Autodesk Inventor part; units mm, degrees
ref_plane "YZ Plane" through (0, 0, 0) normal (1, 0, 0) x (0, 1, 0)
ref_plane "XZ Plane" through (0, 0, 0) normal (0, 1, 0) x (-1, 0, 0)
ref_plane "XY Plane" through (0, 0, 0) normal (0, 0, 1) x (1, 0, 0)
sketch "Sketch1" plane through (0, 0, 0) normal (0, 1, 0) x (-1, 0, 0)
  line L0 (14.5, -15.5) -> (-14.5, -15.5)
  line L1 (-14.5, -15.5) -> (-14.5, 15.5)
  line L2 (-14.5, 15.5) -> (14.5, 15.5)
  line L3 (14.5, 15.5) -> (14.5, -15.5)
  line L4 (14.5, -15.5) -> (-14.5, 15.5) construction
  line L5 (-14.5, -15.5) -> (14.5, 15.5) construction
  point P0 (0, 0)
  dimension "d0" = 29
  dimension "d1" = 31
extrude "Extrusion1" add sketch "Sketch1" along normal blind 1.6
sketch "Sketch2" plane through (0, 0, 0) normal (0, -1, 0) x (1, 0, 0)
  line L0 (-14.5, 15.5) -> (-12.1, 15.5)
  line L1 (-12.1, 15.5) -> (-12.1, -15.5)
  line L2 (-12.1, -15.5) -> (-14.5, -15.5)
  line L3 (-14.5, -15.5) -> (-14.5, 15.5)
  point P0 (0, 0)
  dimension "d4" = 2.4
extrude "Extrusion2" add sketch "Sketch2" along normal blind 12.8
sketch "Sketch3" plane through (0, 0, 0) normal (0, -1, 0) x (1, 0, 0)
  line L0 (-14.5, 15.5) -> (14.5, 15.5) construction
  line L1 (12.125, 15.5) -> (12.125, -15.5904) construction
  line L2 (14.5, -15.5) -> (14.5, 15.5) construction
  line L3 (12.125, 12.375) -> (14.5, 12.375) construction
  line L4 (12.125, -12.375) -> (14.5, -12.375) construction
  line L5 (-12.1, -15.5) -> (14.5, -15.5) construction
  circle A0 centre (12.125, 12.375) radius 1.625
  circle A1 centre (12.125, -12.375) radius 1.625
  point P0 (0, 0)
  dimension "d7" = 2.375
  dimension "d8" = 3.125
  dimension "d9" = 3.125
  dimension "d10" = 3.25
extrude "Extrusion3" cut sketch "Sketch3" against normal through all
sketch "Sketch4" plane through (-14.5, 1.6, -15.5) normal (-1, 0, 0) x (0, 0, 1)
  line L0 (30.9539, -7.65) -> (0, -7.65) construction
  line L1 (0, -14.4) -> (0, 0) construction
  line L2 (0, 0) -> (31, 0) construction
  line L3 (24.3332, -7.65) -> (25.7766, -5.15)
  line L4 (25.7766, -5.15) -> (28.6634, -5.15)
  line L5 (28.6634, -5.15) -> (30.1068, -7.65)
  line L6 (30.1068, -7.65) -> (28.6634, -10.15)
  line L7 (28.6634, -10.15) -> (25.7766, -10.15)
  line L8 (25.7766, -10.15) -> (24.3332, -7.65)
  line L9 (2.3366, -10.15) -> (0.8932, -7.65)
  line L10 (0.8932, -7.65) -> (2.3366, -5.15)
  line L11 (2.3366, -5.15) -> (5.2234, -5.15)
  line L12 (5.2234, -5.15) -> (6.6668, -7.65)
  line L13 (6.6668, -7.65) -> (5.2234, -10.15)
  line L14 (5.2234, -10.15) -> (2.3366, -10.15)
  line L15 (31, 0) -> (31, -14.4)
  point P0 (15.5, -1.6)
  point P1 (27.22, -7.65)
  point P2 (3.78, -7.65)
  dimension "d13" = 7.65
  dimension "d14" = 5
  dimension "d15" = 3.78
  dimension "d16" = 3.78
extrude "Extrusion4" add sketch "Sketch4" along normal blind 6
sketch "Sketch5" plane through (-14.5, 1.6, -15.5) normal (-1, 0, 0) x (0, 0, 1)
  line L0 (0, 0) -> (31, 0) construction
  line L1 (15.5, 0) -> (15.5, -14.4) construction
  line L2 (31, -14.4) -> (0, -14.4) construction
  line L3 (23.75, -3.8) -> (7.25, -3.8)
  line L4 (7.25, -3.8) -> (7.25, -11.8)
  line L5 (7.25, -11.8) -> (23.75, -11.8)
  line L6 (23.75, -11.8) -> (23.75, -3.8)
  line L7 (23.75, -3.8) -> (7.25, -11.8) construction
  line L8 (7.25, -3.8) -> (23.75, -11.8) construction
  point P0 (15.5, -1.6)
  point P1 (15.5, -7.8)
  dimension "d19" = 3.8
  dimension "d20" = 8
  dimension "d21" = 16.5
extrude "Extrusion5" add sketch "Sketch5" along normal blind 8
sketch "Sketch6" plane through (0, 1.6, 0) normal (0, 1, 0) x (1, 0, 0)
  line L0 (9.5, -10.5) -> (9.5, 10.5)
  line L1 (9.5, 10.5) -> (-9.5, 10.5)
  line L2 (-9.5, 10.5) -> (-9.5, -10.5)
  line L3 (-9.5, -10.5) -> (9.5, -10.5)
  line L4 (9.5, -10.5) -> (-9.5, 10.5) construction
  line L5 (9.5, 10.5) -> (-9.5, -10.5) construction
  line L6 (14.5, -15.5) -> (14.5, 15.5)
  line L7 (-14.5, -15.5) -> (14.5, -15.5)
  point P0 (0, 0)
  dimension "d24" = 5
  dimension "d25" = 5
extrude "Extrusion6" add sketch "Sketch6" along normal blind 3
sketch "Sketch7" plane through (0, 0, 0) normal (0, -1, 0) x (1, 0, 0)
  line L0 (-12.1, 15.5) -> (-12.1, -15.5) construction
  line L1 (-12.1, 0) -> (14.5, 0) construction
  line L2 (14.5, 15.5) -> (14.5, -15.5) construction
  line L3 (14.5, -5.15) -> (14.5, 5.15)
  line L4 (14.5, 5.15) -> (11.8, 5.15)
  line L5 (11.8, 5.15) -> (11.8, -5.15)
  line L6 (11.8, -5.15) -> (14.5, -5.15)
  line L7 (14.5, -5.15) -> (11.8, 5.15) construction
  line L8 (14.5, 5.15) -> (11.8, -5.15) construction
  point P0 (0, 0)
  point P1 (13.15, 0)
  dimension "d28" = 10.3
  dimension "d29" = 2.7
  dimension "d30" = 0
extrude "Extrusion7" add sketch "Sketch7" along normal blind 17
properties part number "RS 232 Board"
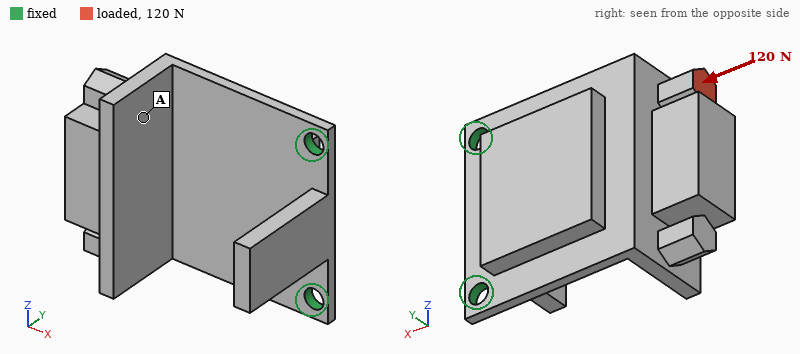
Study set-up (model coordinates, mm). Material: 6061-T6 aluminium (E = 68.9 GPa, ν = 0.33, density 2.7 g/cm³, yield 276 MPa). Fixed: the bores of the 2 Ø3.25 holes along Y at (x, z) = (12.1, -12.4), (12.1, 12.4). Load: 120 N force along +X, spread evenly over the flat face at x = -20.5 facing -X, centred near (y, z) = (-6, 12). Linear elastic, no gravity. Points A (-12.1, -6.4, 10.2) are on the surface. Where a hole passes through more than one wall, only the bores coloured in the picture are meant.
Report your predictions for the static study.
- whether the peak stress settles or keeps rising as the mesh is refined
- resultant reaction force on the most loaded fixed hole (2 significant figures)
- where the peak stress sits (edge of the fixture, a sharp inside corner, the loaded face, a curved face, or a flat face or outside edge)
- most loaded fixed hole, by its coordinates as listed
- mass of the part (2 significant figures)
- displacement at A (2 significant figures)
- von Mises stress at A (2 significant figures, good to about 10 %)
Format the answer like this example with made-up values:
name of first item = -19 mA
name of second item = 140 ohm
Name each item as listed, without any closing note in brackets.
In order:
whether the peak stress settles or keeps rising as the mesh is refined = keeps rising
resultant reaction force on the most loaded fixed hole = 120 N
where the peak stress sits = edge of the fixture
most loaded fixed hole, by its coordinates as listed = (12.1, 12.4)
mass of the part = 14 g
displacement at A = 0.16 mm
von Mises stress at A = 14 MPa
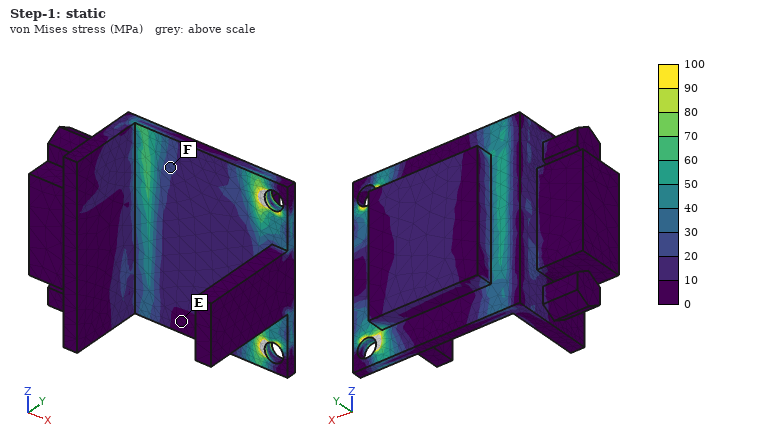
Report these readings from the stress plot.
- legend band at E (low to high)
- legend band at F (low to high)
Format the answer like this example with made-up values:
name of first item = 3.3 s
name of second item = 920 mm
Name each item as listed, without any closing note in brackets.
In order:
legend band at E = 0 to 10 MPa
legend band at F = 20 to 30 MPa
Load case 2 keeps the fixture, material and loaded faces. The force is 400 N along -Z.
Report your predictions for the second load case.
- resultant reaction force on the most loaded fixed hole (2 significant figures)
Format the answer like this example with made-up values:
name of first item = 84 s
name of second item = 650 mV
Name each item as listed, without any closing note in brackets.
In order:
resultant reaction force on the most loaded fixed hole = 560 N
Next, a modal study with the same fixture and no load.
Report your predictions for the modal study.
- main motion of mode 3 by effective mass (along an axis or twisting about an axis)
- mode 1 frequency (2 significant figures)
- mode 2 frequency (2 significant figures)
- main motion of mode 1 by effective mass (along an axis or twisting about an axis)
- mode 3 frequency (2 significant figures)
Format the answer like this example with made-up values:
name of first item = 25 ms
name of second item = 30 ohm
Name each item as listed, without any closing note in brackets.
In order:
main motion of mode 3 by effective mass = along Z
mode 1 frequency = 800 Hz
mode 2 frequency = 3400 Hz
main motion of mode 1 by effective mass = along Y
mode 3 frequency = 3600 Hz
